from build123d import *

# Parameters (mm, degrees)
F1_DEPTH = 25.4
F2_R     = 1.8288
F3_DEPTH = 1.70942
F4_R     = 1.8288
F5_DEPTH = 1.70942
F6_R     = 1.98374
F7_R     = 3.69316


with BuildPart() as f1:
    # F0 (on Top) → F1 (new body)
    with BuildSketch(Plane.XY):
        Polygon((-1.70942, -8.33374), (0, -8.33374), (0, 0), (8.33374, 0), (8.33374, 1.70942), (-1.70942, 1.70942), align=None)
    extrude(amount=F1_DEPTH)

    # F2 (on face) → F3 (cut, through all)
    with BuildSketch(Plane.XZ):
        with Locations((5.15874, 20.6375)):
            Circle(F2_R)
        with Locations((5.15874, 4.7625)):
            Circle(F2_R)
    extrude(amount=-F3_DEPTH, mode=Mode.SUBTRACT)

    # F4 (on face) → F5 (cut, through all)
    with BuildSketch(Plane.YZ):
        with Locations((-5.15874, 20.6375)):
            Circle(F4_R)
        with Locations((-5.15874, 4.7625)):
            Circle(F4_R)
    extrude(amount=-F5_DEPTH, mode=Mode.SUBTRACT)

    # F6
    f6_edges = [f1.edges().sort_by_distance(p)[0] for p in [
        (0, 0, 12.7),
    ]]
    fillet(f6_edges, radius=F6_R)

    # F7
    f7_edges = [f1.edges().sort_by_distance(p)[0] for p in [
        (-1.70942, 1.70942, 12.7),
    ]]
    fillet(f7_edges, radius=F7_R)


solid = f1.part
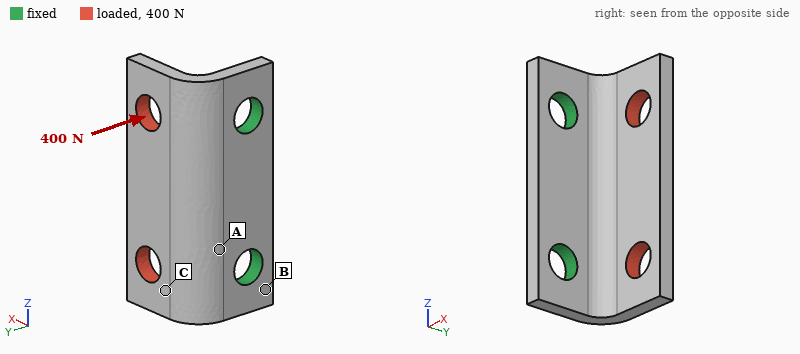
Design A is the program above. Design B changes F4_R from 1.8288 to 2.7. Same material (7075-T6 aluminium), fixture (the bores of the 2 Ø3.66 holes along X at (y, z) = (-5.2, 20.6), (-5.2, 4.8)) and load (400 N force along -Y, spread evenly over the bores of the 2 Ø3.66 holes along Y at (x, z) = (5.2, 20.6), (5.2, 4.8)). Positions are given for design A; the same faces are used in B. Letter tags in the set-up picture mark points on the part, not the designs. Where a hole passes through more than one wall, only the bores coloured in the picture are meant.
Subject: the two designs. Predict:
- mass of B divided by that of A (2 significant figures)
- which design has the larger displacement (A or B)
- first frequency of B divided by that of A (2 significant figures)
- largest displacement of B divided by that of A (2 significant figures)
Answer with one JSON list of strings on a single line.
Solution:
["0.94", "A", "1.1", "0.82"]
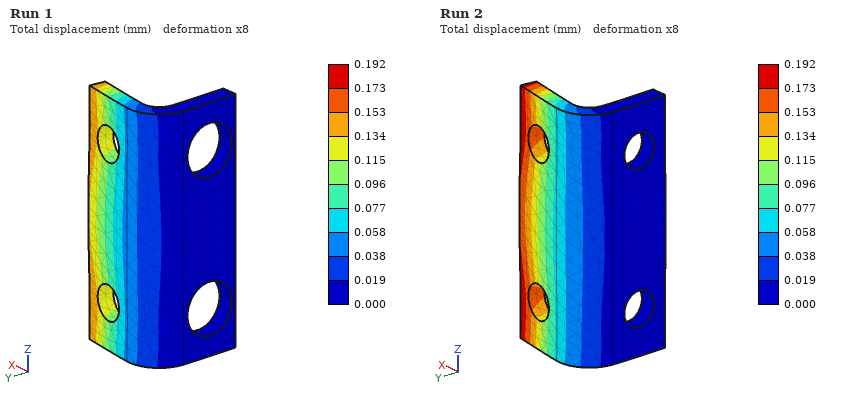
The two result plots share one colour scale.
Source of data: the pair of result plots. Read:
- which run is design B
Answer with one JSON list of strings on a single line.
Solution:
["Run 1"]
